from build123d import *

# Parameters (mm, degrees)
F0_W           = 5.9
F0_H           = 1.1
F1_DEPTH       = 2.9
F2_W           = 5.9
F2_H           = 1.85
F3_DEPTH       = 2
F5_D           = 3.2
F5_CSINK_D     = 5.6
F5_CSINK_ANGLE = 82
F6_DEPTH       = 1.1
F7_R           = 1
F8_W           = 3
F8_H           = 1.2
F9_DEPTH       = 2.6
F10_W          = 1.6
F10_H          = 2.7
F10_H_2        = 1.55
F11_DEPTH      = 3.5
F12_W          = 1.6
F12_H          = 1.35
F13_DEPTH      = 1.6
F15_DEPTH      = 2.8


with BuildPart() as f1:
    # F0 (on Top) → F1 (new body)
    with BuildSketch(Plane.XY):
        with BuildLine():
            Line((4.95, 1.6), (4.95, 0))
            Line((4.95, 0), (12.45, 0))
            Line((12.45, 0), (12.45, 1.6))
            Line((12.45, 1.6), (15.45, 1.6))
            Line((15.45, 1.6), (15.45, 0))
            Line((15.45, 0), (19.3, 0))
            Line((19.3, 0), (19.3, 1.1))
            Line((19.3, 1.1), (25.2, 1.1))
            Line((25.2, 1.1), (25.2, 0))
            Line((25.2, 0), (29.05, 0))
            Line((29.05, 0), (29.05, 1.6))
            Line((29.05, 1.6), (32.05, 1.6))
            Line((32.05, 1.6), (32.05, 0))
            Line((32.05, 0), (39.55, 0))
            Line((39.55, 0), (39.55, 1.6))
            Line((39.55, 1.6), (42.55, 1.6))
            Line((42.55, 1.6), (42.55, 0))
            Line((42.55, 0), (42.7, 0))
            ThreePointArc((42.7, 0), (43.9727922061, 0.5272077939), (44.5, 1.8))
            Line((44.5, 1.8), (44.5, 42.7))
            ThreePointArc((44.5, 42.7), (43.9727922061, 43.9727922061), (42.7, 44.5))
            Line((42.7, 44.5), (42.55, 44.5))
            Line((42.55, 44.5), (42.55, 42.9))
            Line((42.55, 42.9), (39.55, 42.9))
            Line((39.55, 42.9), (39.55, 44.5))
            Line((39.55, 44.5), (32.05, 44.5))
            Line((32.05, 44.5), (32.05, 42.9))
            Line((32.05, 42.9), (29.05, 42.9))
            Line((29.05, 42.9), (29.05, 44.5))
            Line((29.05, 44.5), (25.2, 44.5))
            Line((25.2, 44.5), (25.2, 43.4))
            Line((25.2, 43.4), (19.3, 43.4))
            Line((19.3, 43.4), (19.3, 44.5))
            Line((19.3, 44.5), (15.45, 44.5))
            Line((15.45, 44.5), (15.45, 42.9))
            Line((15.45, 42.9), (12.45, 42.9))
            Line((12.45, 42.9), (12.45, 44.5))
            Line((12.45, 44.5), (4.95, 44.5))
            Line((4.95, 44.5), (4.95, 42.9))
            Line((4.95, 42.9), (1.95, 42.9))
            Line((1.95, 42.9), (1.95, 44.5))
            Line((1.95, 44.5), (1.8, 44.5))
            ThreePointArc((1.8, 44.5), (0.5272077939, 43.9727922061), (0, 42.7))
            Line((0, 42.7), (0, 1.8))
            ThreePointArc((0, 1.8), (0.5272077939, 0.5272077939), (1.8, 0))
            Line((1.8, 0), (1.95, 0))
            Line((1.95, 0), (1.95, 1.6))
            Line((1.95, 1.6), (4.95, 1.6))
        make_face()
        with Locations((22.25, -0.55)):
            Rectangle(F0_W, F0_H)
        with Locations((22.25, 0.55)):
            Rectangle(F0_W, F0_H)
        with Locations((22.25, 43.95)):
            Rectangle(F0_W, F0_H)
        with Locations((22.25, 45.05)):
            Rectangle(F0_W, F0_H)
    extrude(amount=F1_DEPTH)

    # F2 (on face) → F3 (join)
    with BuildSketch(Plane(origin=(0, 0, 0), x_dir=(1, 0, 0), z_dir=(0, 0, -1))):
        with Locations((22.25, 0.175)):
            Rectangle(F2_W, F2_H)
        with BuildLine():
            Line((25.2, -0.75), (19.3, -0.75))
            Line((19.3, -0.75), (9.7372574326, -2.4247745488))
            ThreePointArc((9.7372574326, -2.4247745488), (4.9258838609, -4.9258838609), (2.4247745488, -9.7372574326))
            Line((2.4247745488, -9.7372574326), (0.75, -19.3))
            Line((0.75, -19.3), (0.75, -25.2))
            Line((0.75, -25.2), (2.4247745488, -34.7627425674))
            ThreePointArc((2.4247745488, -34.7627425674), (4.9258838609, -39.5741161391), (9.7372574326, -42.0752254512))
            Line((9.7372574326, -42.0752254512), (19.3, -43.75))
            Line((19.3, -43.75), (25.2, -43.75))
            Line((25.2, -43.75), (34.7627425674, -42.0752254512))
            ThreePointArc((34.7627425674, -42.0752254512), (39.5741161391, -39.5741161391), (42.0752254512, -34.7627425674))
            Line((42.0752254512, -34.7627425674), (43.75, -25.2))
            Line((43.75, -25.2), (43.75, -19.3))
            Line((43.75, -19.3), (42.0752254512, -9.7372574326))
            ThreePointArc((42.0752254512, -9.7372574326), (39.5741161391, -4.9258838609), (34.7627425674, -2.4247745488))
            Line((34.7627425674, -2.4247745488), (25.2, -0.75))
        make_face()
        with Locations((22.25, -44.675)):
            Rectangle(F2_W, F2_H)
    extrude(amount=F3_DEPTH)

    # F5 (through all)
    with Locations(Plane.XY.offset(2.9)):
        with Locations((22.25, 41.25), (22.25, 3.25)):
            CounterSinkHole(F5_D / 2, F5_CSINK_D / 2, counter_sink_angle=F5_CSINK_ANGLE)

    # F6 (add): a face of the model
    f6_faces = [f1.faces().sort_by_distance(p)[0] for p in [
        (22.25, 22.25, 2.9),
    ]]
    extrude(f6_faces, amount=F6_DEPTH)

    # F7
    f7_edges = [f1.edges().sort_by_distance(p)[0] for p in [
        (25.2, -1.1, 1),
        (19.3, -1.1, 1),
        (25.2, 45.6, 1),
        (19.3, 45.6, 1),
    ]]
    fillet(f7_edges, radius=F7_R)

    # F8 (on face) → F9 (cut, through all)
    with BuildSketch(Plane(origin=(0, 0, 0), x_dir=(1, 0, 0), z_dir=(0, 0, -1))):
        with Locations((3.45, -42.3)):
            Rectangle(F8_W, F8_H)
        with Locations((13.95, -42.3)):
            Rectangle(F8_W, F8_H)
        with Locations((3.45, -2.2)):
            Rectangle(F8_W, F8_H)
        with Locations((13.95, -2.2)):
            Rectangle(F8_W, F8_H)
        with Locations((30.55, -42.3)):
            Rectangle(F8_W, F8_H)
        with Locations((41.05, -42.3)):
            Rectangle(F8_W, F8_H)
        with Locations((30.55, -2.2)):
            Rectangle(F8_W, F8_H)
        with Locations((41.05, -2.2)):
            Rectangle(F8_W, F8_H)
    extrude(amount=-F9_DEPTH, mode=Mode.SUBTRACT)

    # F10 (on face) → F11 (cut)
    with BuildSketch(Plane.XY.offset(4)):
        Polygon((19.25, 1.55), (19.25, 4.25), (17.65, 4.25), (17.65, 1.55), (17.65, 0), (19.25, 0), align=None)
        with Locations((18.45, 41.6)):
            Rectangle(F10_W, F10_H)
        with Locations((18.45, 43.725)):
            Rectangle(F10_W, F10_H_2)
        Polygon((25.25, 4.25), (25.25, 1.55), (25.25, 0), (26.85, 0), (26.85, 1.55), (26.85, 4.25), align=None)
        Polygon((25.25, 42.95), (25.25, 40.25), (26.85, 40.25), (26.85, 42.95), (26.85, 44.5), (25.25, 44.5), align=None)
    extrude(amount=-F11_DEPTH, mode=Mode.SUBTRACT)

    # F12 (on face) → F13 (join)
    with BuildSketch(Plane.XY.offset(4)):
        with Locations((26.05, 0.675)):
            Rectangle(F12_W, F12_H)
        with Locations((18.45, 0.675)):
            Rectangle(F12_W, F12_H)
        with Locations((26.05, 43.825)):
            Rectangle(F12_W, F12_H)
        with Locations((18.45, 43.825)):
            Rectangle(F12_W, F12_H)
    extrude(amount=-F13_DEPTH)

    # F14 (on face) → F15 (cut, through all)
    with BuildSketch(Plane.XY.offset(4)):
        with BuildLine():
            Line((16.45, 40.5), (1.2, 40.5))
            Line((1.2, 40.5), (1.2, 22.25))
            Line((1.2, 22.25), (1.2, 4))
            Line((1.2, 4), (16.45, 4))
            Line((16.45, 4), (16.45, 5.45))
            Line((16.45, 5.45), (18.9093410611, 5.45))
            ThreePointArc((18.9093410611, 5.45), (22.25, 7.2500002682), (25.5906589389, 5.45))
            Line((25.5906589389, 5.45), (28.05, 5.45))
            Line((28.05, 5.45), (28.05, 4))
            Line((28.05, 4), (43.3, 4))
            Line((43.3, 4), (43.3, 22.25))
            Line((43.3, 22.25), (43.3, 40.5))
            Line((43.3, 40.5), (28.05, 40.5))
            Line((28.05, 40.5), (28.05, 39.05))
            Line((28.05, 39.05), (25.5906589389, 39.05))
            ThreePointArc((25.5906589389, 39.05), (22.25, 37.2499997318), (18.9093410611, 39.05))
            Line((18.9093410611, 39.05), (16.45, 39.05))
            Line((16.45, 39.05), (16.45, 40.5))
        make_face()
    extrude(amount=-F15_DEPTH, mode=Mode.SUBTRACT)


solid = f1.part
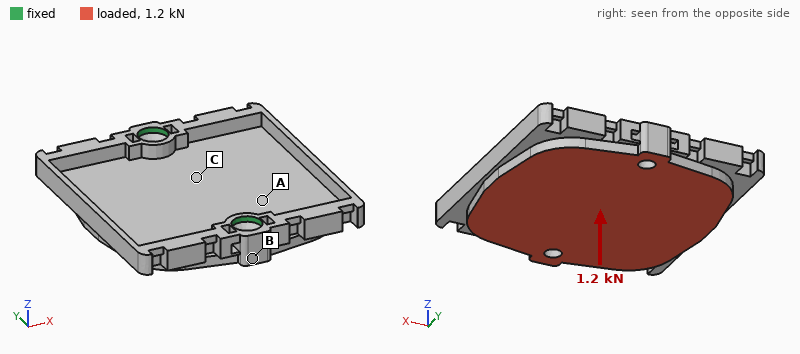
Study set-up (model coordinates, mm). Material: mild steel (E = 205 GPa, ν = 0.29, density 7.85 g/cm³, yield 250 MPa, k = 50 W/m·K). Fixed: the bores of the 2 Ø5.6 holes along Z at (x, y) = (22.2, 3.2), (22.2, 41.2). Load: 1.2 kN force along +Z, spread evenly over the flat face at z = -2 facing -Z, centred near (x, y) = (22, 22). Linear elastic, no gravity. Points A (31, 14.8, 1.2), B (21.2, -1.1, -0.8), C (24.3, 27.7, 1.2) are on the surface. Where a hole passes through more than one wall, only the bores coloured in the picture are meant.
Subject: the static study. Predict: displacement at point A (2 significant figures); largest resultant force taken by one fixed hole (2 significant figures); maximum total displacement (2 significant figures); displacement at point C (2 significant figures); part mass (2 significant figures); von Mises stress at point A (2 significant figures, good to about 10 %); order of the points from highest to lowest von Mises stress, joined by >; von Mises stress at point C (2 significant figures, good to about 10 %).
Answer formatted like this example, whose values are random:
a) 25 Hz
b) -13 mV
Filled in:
a) 11 µm
b) 700 N
c) 24 µm
d) 8.9 µm
e) 52 g
f) 20 MPa
g) C > A > B
h) 33 MPa
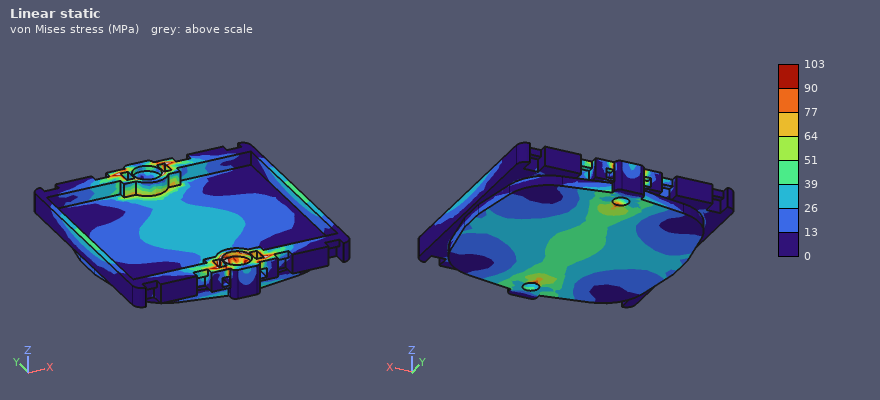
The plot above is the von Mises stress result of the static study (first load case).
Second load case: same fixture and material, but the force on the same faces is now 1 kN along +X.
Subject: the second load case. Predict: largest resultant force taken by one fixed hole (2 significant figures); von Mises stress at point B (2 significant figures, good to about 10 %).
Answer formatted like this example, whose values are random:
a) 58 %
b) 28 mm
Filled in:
a) 500 N
b) 13 MPa
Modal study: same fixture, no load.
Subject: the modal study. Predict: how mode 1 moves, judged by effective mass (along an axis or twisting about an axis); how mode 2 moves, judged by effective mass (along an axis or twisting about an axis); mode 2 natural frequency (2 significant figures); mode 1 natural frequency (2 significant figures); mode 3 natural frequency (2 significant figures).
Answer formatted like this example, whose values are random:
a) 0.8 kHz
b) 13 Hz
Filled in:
a) twisting about Y
b) along Z
c) 6300 Hz
d) 4300 Hz
e) 8300 Hz
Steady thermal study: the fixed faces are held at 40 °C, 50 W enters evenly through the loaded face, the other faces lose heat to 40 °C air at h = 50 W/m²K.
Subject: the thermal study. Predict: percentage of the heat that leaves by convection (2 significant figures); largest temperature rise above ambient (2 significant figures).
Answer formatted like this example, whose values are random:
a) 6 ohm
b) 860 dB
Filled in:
a) 24 %
b) 77 K
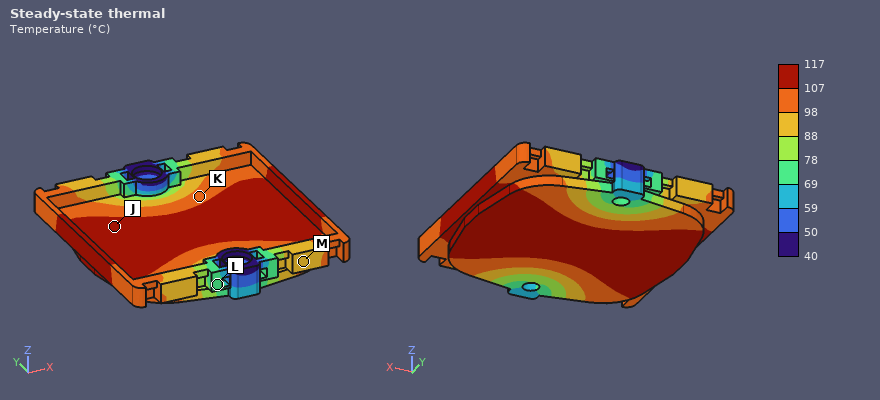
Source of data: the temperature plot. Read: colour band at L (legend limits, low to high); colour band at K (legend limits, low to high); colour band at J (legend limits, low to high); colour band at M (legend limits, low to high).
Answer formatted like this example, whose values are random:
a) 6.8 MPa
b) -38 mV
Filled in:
a) 69 to 78 °C
b) 98 to 107 °C
c) 107 to 117 °C
d) 88 to 98 °C
